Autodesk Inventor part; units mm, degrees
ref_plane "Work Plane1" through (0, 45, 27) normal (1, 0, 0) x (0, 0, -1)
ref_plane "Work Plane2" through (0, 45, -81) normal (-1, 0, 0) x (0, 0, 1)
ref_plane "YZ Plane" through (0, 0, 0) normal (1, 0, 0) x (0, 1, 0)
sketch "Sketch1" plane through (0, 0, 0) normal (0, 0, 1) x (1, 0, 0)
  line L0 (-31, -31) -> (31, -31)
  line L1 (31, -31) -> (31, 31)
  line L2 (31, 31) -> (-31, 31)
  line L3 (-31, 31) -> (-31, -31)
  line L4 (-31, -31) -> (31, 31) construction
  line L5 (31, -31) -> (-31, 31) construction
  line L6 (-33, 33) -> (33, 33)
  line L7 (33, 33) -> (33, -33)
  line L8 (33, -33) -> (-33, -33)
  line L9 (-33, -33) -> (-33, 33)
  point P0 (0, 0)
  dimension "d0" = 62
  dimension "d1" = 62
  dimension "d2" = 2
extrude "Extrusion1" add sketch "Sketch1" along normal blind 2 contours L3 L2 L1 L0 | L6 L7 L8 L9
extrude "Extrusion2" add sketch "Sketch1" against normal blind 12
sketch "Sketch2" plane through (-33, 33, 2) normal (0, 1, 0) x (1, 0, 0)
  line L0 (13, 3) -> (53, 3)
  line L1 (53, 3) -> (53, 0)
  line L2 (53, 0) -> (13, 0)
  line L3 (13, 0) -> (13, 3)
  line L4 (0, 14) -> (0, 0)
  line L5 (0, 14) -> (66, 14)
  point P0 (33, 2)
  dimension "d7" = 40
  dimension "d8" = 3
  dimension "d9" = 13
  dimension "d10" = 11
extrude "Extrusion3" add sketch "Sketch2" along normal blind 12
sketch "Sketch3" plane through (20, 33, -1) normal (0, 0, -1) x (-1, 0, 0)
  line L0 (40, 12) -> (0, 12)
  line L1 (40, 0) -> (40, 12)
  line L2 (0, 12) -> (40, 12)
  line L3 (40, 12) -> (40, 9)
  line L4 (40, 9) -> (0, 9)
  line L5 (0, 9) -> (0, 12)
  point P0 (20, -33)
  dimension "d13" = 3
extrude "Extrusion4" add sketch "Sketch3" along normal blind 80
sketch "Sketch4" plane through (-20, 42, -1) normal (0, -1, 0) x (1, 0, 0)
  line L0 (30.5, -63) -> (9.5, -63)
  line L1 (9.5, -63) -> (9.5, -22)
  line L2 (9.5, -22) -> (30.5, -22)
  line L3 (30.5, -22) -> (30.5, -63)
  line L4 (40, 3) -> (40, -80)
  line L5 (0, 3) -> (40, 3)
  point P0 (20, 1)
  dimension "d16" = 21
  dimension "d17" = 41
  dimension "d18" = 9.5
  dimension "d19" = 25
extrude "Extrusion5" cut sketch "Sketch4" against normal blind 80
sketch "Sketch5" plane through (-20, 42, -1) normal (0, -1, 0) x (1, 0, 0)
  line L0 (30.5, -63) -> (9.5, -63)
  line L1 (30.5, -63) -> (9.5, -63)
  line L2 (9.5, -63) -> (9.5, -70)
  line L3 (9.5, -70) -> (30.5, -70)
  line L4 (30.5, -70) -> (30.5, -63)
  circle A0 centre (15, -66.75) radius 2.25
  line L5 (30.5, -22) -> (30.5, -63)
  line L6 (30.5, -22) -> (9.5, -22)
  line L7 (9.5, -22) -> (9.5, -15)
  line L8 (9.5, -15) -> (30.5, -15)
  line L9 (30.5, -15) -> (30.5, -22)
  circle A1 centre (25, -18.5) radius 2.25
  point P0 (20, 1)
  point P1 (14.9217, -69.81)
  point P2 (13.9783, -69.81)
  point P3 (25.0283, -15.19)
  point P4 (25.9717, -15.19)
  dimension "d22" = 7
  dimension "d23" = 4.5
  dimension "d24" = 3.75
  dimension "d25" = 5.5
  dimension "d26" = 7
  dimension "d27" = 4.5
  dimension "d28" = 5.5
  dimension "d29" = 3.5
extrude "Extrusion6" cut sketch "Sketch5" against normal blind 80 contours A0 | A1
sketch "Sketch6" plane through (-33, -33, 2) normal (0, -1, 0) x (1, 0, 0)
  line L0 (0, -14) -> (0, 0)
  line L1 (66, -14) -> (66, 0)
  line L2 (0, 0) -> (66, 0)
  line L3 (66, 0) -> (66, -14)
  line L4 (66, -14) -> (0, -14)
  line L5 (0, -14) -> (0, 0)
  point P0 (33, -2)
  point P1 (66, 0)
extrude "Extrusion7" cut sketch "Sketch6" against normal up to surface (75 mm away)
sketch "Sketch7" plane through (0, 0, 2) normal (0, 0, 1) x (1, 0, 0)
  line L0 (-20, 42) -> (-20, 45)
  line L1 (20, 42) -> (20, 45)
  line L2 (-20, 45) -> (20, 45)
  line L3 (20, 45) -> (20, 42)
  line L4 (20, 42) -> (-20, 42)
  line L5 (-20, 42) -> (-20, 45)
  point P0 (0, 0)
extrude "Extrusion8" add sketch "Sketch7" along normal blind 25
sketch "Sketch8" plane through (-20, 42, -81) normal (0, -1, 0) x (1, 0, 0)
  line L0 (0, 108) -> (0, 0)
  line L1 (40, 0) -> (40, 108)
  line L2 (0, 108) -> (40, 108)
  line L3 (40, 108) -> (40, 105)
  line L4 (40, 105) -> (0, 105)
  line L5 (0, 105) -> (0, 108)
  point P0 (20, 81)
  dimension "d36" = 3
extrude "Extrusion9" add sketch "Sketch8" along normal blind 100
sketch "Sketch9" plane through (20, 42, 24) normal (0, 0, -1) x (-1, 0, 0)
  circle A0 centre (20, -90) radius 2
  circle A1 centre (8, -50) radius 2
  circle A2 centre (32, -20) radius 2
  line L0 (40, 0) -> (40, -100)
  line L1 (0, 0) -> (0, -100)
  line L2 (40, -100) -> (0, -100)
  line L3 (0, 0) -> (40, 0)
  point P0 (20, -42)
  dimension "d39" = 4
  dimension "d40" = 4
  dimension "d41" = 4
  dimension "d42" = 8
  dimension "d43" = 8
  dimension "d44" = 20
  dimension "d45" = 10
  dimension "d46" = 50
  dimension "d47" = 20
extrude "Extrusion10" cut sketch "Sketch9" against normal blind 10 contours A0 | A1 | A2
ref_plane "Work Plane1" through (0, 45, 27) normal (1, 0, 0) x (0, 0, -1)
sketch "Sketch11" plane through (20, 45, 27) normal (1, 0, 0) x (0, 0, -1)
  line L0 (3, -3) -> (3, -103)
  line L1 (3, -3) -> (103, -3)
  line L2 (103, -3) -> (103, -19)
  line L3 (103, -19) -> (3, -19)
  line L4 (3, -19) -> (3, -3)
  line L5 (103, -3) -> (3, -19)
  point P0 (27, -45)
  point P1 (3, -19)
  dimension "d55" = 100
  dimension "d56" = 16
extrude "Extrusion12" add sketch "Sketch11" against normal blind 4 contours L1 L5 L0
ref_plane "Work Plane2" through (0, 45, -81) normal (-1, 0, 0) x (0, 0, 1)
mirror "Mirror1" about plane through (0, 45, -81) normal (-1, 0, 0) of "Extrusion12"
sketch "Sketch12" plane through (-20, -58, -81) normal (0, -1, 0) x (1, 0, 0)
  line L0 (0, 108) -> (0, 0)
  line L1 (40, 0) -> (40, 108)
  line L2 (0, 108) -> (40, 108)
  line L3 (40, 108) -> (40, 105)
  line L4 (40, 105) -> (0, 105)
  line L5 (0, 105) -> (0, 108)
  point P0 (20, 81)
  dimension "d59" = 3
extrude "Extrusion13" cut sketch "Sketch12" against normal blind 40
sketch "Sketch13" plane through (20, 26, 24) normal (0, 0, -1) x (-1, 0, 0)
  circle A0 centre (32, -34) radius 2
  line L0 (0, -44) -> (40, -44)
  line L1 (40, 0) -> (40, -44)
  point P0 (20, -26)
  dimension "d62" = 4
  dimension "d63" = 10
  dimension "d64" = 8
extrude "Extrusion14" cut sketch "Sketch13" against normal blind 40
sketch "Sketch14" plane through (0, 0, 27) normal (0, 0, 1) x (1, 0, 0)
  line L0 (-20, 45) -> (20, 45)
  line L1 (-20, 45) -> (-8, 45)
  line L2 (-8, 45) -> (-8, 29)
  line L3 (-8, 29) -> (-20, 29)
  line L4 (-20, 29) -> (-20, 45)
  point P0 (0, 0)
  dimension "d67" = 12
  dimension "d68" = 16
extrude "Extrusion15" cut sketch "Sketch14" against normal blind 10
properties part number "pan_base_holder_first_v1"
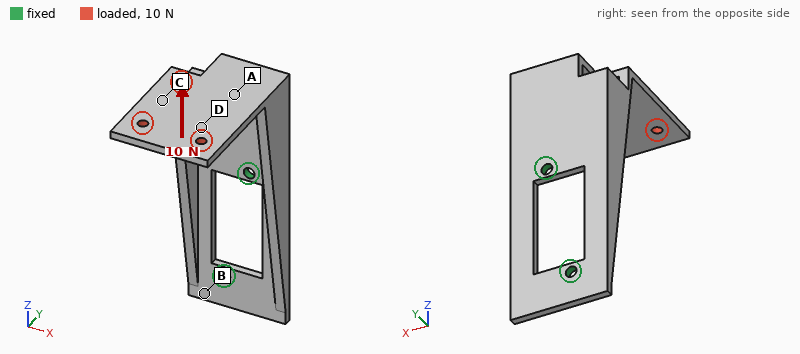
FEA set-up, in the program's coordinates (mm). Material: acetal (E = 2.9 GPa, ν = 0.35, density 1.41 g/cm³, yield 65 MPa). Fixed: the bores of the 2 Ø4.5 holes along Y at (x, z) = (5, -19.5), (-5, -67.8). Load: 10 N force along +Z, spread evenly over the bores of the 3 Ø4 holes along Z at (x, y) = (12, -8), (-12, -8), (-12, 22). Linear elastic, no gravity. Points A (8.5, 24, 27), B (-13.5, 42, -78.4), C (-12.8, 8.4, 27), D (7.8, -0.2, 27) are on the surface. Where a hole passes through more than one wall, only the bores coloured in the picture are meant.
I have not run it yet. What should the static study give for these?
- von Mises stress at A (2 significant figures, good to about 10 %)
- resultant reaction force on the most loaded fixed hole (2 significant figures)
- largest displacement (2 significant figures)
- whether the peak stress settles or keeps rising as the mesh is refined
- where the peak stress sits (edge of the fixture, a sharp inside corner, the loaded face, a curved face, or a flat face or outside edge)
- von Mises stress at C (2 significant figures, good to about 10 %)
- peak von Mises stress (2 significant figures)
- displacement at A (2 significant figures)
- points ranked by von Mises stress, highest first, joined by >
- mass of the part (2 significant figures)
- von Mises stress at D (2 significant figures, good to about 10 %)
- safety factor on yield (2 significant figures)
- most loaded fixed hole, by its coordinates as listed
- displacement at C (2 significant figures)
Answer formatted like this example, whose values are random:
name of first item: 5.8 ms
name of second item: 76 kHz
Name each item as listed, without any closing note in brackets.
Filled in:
von Mises stress at A: 4.1 MPa
resultant reaction force on the most loaded fixed hole: 15 N
largest displacement: 1.4 mm
whether the peak stress settles or keeps rising as the mesh is refined: settles
where the peak stress sits: a flat face or outside edge
von Mises stress at C: 1.9 MPa
peak von Mises stress: 10.0 MPa
displacement at A: 0.27 mm
points ranked by von Mises stress, highest first, joined by >: A > C > D > B
mass of the part: 32 g
von Mises stress at D: 1.2 MPa
safety factor on yield: 6.5
most loaded fixed hole, by its coordinates as listed: (-5, -67.8)
displacement at C: 0.59 mm
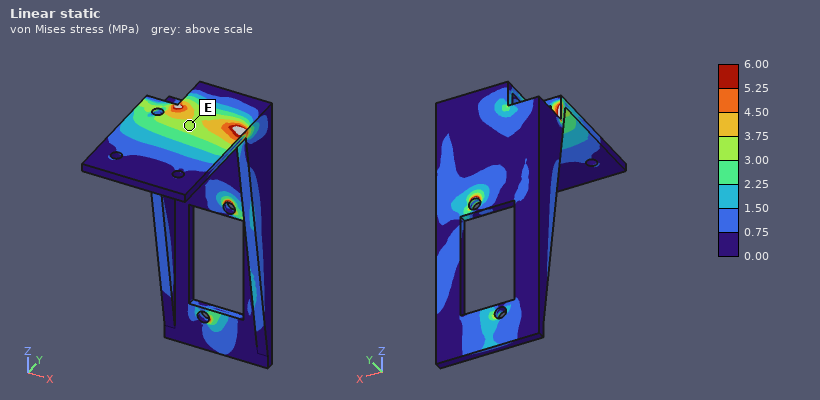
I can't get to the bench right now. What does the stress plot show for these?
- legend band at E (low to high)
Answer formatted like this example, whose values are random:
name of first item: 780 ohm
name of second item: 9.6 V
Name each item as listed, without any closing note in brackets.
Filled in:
legend band at E: 3.00 to 3.75 MPa
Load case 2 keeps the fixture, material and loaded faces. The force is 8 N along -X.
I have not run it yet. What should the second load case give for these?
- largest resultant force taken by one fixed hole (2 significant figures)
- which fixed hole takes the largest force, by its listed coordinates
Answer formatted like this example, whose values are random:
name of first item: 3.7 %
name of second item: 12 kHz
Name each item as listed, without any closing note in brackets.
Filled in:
largest resultant force taken by one fixed hole: 13 N
which fixed hole takes the largest force, by its listed coordinates: (5, -19.5)
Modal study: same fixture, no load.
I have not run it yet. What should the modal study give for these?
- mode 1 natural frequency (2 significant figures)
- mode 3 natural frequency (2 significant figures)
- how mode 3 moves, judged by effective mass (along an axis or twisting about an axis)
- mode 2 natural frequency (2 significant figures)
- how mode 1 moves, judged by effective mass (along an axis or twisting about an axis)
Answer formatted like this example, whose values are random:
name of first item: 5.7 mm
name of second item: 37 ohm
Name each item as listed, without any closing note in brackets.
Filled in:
mode 1 natural frequency: 160 Hz
mode 3 natural frequency: 350 Hz
how mode 3 moves, judged by effective mass: along Y
mode 2 natural frequency: 200 Hz
how mode 1 moves, judged by effective mass: along X
